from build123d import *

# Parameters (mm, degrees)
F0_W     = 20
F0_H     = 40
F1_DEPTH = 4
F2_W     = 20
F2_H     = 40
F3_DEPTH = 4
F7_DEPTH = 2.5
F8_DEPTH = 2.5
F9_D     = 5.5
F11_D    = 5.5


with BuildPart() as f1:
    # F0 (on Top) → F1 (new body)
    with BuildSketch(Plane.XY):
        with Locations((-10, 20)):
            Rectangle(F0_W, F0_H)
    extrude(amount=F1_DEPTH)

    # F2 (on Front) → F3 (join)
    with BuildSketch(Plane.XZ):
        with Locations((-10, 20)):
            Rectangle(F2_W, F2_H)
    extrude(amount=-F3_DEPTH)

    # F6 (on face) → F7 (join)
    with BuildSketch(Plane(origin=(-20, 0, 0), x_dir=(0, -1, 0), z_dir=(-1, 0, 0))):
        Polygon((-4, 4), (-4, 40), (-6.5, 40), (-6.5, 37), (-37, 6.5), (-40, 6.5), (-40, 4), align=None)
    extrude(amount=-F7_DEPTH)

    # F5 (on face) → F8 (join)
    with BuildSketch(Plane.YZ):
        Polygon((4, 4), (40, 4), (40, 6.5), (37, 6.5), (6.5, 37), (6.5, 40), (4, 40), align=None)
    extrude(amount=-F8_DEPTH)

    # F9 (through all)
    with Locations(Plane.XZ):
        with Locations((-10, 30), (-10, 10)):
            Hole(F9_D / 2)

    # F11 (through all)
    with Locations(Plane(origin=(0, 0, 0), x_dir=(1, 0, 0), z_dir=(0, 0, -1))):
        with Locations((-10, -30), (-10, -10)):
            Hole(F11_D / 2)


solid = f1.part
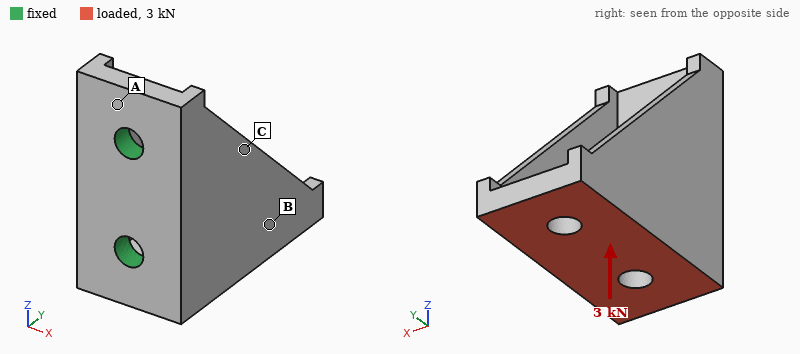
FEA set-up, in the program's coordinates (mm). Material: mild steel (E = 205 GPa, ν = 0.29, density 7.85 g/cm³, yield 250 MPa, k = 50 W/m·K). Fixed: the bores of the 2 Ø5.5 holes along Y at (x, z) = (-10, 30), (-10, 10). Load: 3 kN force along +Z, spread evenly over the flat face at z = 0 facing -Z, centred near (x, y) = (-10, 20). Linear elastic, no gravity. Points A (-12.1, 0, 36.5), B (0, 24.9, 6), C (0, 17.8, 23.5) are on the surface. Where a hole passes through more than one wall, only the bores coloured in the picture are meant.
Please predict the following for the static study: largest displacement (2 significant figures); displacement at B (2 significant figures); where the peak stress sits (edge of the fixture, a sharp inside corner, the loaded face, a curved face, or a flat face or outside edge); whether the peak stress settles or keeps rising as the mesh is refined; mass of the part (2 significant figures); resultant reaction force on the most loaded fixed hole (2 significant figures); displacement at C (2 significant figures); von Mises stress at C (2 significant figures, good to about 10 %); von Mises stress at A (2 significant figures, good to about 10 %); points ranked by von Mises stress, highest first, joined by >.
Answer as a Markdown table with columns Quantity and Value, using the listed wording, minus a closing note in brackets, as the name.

| Quantity | Value |
|---|---|
| largest displacement | 43 µm |
| displacement at B | 21 µm |
| where the peak stress sits | edge of the fixture |
| whether the peak stress settles or keeps rising as the mesh is refined | keeps rising |
| mass of the part | 70 g |
| resultant reaction force on the most loaded fixed hole | 2.6 kN |
| displacement at C | 16 µm |
| von Mises stress at C | 45 MPa |
| von Mises stress at A | 91 MPa |
| points ranked by von Mises stress, highest first, joined by > | A > C > B |
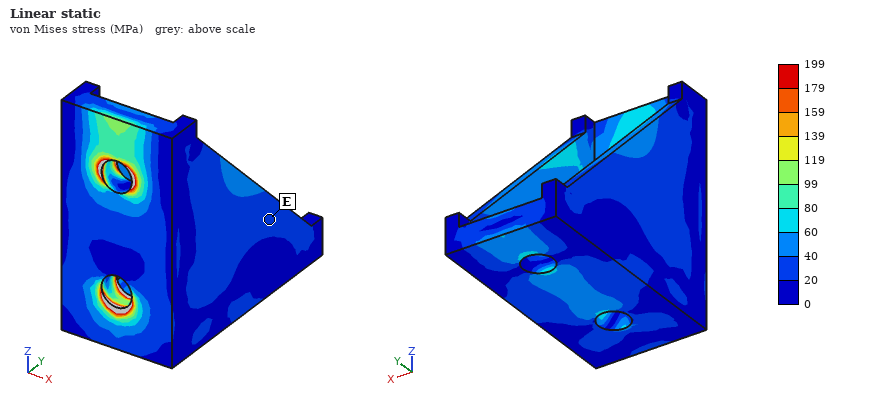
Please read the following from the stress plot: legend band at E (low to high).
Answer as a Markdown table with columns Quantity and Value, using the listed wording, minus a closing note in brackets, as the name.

| Quantity | Value |
|---|---|
| legend band at E | 20 to 40 MPa |
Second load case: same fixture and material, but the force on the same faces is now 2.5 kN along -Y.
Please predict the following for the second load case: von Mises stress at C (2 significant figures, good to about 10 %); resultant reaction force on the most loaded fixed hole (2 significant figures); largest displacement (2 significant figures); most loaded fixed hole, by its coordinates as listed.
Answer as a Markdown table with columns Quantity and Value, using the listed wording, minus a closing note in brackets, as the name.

| Quantity | Value |
|---|---|
| von Mises stress at C | 23 MPa |
| resultant reaction force on the most loaded fixed hole | 3.2 kN |
| largest displacement | 27 µm |
| most loaded fixed hole, by its coordinates as listed | (-10, 10) |
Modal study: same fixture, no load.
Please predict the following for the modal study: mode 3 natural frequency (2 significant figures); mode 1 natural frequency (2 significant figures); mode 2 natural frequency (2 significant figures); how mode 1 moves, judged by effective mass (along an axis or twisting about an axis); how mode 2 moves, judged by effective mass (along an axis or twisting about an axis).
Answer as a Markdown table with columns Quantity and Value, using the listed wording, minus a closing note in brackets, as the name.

| Quantity | Value |
|---|---|
| mode 3 natural frequency | 11 kHz |
| mode 1 natural frequency | 3700 Hz |
| mode 2 natural frequency | 8100 Hz |
| how mode 1 moves, judged by effective mass | along X |
| how mode 2 moves, judged by effective mass | along Z |
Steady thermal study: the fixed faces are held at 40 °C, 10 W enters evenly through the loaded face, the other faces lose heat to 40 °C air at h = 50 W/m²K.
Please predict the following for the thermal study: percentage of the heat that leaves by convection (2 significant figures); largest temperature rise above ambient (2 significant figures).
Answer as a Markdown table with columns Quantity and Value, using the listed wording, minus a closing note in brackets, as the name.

| Quantity | Value |
|---|---|
| percentage of the heat that leaves by convection | 26 % |
| largest temperature rise above ambient | 25 K |
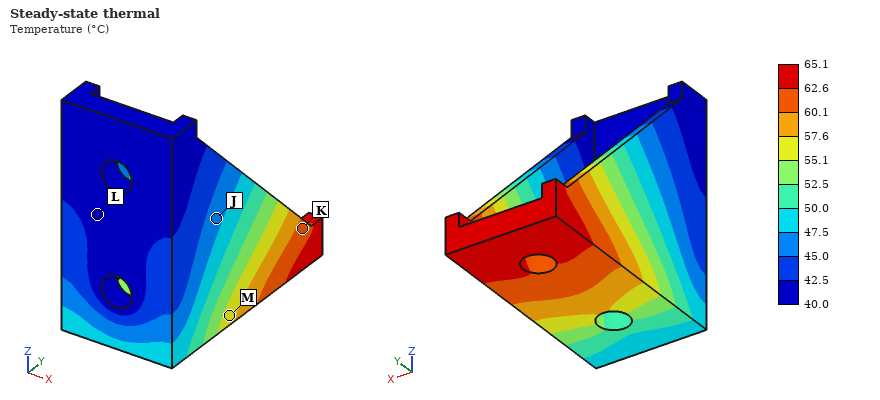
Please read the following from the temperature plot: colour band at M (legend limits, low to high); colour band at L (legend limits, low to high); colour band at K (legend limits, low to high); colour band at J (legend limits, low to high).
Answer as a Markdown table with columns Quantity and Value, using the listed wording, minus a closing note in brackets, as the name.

| Quantity | Value |
|---|---|
| colour band at M | 55.1 to 57.6 °C |
| colour band at L | 40.0 to 42.5 °C |
| colour band at K | 60.1 to 62.6 °C |
| colour band at J | 45.0 to 47.5 °C |
